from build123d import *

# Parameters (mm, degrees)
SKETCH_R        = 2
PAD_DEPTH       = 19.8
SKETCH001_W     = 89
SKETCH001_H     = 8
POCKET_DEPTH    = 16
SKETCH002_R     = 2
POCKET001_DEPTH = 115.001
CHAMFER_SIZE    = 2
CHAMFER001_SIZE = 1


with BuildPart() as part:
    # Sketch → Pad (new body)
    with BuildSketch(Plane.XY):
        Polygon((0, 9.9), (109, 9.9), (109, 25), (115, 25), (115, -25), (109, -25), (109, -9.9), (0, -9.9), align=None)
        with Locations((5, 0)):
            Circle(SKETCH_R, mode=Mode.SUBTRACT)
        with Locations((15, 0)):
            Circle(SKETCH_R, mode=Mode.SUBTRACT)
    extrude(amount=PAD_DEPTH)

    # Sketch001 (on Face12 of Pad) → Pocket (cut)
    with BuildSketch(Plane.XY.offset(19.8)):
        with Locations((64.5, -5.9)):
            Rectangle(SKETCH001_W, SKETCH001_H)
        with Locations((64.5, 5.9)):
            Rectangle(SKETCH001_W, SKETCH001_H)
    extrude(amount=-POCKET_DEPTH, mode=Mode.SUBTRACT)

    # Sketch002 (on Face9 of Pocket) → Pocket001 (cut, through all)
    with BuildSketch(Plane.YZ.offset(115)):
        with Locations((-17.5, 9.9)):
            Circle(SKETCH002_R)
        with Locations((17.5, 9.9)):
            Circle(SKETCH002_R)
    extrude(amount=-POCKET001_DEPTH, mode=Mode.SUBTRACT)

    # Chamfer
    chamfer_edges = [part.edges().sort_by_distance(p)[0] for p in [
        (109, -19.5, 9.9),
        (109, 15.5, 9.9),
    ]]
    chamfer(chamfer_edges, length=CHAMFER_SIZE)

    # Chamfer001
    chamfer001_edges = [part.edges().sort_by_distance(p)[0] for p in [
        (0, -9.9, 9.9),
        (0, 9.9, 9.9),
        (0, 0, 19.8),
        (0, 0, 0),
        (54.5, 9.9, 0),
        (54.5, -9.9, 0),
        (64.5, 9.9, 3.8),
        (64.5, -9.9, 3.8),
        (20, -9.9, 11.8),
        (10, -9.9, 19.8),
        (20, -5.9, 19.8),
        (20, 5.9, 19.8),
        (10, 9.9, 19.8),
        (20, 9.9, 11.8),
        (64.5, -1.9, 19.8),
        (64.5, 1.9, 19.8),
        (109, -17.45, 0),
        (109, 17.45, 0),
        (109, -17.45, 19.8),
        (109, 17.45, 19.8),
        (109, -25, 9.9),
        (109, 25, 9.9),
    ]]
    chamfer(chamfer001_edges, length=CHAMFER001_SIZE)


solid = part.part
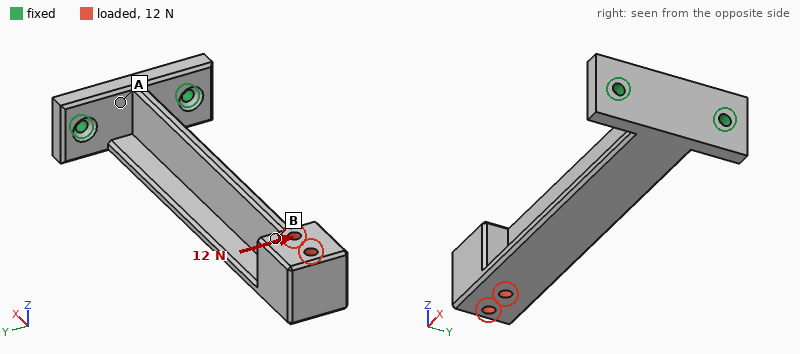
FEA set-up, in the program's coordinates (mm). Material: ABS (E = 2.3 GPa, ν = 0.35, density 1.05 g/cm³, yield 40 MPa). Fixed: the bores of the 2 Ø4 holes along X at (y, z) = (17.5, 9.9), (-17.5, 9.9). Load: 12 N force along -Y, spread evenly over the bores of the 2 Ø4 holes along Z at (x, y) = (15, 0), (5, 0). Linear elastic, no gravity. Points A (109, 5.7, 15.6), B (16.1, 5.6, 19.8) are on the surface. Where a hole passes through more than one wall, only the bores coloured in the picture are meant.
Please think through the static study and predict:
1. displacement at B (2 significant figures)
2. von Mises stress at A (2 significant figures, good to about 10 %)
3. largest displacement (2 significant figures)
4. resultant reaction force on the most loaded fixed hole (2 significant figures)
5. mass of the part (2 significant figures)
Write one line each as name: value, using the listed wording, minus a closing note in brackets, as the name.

displacement at B: 1.2 mm
von Mises stress at A: 1.3 MPa
largest displacement: 1.4 mm
resultant reaction force on the most loaded fixed hole: 43 N
mass of the part: 26 g
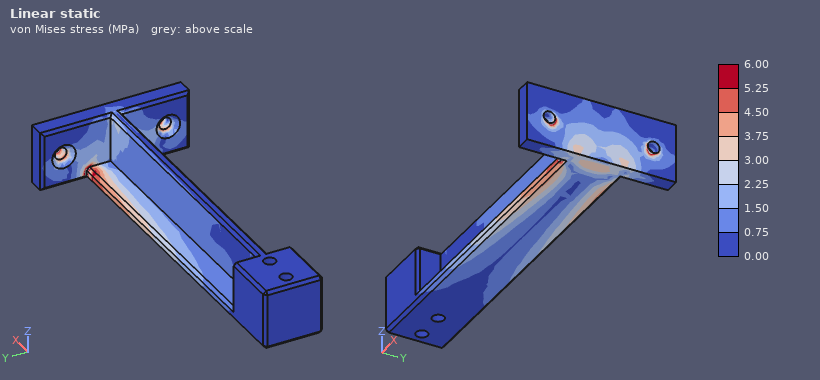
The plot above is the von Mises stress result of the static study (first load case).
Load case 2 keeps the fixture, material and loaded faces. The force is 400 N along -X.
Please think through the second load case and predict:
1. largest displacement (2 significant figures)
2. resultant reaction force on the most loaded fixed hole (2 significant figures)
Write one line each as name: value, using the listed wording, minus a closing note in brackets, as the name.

largest displacement: 1.4 mm
resultant reaction force on the most loaded fixed hole: 230 N
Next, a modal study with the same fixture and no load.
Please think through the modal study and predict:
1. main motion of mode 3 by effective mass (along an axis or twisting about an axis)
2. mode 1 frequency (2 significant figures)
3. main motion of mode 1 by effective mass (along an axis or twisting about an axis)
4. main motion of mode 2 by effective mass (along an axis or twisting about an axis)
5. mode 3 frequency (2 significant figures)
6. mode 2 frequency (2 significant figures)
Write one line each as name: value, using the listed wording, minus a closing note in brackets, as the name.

main motion of mode 3 by effective mass: twisting about X
mode 1 frequency: 150 Hz
main motion of mode 1 by effective mass: along Z
main motion of mode 2 by effective mass: along Y
mode 3 frequency: 500 Hz
mode 2 frequency: 160 Hz
